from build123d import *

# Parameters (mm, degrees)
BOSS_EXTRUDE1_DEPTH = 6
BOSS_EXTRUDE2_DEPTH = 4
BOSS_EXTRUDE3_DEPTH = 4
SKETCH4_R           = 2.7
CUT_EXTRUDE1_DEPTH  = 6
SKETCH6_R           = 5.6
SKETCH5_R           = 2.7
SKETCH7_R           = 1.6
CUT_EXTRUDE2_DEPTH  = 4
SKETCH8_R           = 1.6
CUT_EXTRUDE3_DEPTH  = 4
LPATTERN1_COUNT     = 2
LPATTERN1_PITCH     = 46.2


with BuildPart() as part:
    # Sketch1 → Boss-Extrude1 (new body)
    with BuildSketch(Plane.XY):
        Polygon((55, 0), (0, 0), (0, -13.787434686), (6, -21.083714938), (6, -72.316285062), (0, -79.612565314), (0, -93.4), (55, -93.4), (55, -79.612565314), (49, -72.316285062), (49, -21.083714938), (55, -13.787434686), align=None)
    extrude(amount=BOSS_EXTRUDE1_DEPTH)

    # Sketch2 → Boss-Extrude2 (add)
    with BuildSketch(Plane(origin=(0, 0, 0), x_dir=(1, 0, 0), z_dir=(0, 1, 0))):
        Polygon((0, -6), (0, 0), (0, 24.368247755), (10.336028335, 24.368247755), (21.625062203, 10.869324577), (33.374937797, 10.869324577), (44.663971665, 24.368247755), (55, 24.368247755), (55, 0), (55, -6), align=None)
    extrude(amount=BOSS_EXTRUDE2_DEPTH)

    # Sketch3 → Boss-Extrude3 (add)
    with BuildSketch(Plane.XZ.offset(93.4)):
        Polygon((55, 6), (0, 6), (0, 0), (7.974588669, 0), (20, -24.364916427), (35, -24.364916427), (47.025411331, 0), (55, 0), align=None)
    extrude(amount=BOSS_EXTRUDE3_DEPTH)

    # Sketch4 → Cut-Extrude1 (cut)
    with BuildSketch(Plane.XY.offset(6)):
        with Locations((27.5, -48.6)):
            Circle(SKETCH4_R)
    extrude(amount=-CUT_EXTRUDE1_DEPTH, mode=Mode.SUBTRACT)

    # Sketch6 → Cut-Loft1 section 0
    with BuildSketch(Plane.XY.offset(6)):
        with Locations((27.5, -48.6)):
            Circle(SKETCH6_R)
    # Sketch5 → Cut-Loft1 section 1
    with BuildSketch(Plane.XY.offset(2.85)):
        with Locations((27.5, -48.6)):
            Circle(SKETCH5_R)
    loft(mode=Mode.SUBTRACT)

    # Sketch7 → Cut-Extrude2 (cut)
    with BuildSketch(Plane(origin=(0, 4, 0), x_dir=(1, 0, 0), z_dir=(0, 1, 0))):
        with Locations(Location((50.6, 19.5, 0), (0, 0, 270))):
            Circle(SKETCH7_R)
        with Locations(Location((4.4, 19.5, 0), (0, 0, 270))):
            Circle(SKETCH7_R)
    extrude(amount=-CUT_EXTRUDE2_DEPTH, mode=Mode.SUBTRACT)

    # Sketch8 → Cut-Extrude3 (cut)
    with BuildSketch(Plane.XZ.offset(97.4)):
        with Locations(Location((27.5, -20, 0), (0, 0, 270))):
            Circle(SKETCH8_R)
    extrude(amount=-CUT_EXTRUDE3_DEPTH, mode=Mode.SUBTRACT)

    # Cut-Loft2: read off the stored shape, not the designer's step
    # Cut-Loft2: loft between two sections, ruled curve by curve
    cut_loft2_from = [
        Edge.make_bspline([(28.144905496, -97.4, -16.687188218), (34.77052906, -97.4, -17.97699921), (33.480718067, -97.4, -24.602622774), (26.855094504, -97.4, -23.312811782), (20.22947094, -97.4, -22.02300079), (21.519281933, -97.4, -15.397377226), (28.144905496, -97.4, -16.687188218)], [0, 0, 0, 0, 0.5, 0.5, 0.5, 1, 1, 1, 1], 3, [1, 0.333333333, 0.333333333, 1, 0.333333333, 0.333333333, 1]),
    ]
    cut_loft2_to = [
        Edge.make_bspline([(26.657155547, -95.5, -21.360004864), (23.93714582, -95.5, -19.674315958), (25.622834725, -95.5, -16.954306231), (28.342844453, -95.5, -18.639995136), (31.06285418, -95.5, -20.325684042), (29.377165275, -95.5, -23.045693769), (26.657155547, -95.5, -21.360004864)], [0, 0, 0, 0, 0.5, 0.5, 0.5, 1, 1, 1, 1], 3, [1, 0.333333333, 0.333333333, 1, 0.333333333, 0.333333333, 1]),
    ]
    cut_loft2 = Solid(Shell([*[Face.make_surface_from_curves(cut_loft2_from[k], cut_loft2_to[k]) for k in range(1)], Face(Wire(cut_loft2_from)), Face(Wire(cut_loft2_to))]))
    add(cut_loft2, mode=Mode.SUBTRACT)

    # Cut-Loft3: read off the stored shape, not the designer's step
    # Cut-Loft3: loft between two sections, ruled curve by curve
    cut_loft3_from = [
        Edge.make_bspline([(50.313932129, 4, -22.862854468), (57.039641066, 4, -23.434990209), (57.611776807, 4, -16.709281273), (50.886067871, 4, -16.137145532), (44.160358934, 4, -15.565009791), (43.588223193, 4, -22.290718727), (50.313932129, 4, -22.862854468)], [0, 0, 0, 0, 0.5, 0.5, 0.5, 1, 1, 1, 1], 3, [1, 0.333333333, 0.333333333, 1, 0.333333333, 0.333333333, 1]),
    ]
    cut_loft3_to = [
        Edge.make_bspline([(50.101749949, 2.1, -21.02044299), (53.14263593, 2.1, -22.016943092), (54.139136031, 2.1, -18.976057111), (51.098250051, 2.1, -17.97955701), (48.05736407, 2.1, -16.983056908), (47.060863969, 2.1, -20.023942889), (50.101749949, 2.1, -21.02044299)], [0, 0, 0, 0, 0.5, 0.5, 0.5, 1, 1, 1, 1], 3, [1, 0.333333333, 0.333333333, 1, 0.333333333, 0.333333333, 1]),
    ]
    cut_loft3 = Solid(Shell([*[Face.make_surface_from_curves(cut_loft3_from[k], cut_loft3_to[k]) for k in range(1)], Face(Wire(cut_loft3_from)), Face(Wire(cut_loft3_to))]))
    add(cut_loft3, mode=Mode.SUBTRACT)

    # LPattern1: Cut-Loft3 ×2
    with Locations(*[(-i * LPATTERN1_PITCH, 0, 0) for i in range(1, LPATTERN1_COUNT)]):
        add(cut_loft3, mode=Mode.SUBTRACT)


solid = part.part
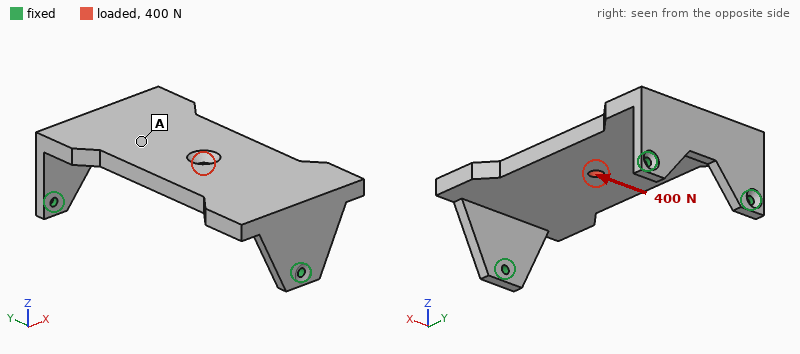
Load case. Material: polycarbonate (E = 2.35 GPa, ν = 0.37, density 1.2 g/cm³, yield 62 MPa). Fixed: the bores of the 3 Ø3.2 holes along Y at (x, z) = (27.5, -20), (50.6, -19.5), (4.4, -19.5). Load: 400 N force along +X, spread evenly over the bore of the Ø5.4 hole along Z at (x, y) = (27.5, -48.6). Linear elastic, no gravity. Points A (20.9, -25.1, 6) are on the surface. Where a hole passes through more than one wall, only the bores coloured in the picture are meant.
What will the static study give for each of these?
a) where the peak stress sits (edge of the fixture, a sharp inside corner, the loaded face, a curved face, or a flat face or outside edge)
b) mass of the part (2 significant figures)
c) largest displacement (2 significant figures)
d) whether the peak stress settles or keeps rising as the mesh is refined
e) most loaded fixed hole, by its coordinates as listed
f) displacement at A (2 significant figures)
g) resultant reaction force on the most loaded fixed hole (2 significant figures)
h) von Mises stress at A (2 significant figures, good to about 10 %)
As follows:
edge of the fixture
43 g
1.3 mm
keeps rising
(27.5, -20)
0.36 mm
190 N
4.3 MPa
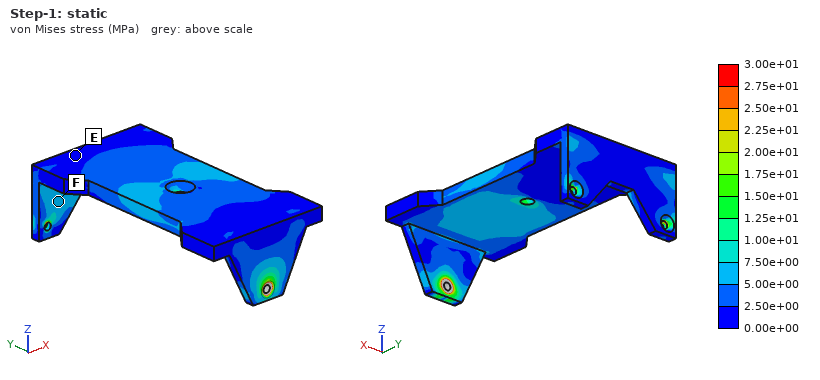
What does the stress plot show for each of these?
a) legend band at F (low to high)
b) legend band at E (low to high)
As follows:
5.00e+00 to 7.50e+00 MPa
0.00e+00 to 2.50e+00 MPa
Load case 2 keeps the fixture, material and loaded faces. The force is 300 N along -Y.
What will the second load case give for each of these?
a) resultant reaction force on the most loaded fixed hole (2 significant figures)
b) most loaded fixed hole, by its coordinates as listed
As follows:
150 N
(27.5, -20)
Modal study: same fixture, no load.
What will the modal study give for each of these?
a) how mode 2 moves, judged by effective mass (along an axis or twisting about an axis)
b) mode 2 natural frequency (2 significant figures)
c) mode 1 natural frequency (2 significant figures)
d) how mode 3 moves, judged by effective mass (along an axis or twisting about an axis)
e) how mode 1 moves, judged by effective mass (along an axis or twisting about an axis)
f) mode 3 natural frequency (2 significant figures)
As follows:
along X
560 Hz
540 Hz
along Z
along Y
600 Hz
